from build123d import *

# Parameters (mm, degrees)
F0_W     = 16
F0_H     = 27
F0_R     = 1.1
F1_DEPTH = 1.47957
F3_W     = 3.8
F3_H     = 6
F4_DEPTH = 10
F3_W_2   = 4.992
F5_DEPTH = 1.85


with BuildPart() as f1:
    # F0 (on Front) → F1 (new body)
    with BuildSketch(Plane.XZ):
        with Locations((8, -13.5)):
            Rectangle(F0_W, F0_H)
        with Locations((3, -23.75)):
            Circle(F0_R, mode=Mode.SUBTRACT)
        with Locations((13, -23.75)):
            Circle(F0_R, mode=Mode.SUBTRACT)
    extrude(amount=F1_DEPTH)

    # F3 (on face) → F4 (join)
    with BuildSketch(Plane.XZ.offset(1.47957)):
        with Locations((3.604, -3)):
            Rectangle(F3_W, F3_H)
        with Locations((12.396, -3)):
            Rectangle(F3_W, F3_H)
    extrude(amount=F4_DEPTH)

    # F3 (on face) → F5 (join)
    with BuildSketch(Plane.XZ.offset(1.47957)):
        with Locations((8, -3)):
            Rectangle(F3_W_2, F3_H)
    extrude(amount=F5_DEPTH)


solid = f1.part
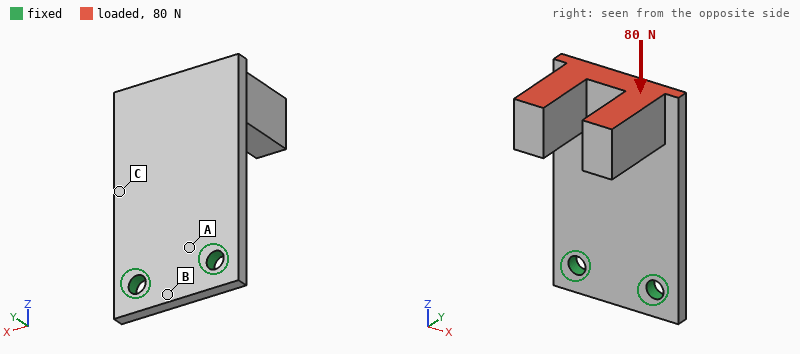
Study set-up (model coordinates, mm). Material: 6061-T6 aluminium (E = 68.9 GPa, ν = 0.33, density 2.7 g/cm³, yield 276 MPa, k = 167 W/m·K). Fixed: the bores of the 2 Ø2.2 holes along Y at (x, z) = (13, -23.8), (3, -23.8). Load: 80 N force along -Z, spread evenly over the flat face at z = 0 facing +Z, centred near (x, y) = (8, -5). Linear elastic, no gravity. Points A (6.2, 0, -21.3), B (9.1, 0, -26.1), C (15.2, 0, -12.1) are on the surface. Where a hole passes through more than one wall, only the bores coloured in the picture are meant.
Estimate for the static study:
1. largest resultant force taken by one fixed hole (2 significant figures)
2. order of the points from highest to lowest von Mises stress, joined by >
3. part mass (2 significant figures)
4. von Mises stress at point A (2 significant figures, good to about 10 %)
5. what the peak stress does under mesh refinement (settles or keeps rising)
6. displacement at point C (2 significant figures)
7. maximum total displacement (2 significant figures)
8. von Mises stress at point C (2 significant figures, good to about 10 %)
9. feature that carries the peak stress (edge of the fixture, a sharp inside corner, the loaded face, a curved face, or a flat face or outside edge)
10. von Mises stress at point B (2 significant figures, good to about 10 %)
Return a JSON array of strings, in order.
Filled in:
["40 N", "C > A > B", "3.1 g", "44 MPa", "keeps rising", "0.067 mm", "0.35 mm", "55 MPa", "edge of the fixture", "9.0 MPa"]
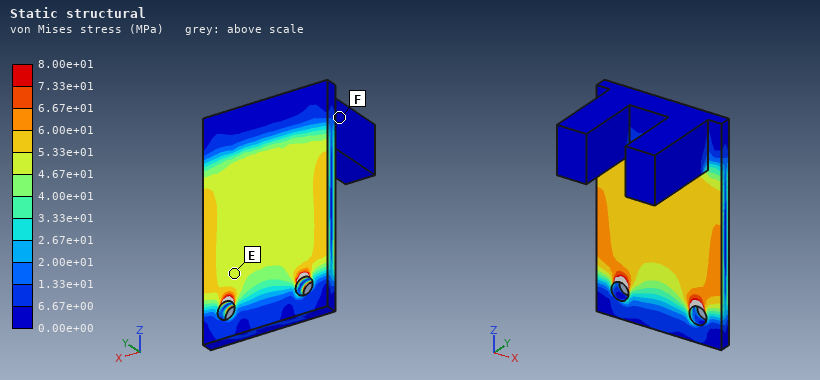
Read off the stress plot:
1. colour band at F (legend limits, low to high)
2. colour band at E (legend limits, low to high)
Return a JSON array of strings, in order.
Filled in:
["0.00e+00 to 6.67e+00 MPa", "4.67e+01 to 5.33e+01 MPa"]
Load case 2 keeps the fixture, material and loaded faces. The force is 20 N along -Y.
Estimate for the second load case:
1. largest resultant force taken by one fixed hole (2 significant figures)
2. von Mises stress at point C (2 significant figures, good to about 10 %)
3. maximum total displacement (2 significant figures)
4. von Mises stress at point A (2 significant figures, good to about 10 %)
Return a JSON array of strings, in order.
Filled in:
["10 N", "43 MPa", "0.33 mm", "58 MPa"]
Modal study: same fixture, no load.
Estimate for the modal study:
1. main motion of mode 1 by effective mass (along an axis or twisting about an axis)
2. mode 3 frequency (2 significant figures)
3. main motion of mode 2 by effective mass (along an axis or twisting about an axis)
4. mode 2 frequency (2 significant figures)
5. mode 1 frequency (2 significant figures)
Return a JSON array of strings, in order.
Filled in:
["along Y", "6100 Hz", "along X", "3100 Hz", "1100 Hz"]
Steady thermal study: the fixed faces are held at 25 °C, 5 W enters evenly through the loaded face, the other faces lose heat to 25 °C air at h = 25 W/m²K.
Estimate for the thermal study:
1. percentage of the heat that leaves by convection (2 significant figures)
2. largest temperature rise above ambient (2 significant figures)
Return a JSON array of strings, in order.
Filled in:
["9.3 %", "25 K"]
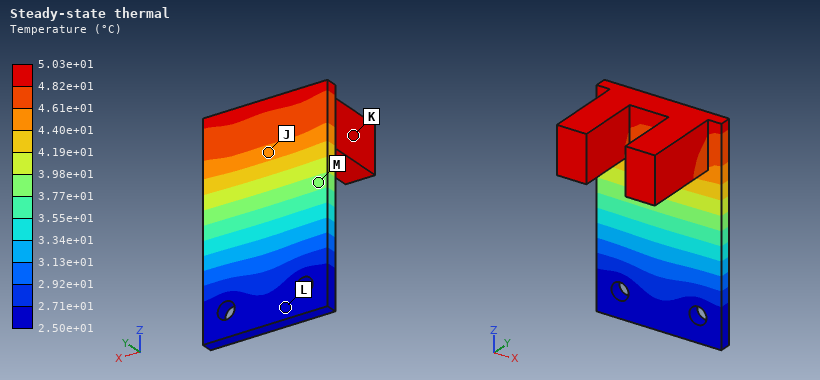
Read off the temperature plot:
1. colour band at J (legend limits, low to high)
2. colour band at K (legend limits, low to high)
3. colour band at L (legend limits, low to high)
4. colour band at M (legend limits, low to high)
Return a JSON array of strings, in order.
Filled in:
["4.40e+01 to 4.61e+01 °C", "4.82e+01 to 5.03e+01 °C", "2.50e+01 to 2.71e+01 °C", "3.77e+01 to 3.98e+01 °C"]
